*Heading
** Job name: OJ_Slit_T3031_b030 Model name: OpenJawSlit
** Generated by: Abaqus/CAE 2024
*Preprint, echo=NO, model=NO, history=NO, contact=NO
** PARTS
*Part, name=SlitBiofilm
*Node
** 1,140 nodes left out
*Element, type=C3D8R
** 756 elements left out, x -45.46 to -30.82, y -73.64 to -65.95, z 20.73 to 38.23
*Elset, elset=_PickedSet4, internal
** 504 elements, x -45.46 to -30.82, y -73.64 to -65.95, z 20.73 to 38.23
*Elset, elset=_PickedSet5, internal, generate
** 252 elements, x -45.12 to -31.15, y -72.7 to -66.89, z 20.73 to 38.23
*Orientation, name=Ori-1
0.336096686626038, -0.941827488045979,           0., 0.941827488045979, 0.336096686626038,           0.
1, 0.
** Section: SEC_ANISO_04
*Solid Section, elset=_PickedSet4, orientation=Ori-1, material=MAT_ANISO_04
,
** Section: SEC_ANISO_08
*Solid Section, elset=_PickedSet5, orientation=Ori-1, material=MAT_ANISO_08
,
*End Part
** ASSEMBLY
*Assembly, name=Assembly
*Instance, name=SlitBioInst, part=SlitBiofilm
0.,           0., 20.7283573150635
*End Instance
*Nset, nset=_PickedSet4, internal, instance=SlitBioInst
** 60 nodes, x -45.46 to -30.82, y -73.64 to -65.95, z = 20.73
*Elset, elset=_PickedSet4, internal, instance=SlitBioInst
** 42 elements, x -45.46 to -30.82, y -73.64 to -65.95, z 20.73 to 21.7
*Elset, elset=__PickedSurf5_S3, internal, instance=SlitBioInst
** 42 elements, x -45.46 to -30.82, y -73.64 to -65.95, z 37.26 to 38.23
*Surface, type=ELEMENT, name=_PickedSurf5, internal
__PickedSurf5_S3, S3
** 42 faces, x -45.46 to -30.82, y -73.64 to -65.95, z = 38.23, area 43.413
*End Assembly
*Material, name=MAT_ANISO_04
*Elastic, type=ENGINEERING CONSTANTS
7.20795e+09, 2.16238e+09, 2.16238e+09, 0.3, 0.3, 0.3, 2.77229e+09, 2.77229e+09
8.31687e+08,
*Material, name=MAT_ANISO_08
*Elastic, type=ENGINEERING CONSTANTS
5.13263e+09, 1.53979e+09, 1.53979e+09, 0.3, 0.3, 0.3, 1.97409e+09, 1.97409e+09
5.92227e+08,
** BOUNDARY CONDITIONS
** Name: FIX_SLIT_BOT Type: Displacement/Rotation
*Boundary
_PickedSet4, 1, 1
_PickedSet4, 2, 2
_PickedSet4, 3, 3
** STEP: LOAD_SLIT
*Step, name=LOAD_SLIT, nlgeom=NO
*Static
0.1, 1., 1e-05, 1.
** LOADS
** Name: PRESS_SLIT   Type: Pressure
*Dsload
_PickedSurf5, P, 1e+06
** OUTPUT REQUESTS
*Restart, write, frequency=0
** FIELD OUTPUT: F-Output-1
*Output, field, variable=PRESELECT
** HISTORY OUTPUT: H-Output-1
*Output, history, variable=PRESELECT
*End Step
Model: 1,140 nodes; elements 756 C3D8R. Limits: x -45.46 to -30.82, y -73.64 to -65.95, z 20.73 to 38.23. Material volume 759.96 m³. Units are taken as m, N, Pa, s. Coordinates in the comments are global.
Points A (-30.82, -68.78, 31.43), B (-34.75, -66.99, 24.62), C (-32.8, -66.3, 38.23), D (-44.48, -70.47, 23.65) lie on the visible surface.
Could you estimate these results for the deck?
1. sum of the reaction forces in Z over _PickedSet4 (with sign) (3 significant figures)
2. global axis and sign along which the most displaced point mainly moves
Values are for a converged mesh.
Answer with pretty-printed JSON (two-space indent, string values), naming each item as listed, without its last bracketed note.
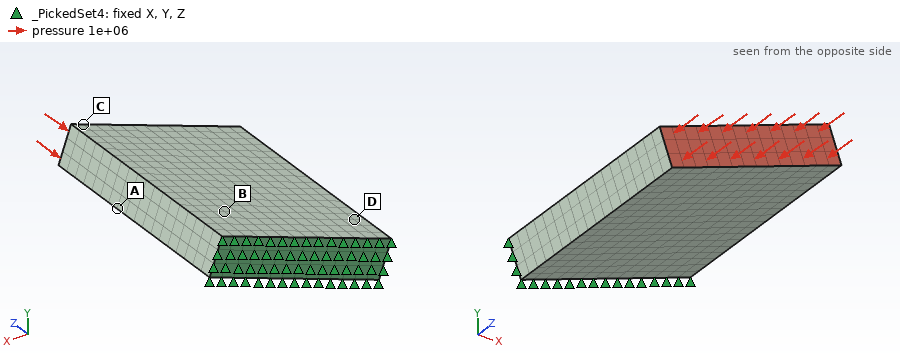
{
  "sum of the reaction forces in Z over _PickedSet4 (with sign)": "4.34e+07 N",
  "global axis and sign along which the most displaced point mainly moves": "-Z"
}
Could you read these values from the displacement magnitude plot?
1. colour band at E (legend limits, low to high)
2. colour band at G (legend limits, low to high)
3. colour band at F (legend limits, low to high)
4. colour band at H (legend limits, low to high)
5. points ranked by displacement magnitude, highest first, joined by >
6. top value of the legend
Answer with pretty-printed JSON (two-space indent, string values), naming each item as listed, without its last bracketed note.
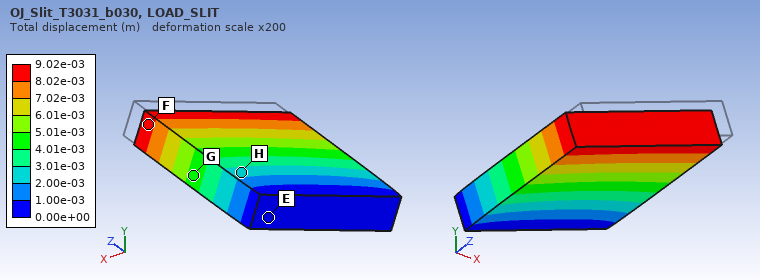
{
  "colour band at E": "0.00e+00 to 1.00e-03 m",
  "colour band at G": "4.01e-03 to 5.01e-03 m",
  "colour band at F": "8.02e-03 to 9.02e-03 m",
  "colour band at H": "2.00e-03 to 3.01e-03 m",
  "points ranked by displacement magnitude, highest first, joined by >": "F > G > H > E",
  "top value of the legend": "9.02e-03 m"
}
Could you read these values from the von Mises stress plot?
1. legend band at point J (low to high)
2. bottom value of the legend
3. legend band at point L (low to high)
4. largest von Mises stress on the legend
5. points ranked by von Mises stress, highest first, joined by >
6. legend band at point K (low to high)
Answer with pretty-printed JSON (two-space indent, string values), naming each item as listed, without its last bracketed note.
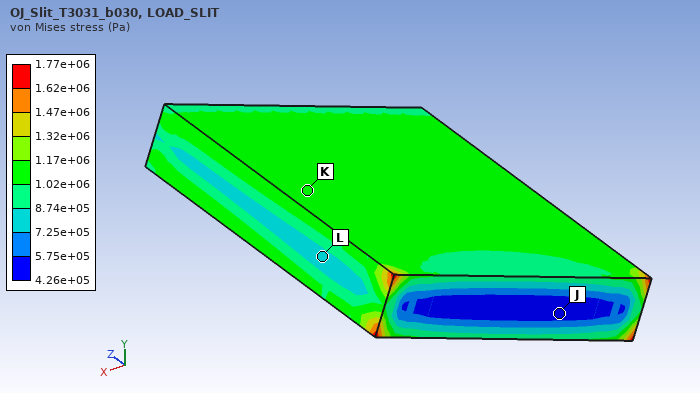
{
  "legend band at point J": "4.26e+05 to 5.75e+05 Pa",
  "bottom value of the legend": "4.26e+05 Pa",
  "legend band at point L": "7.25e+05 to 8.74e+05 Pa",
  "largest von Mises stress on the legend": "1.77e+06 Pa",
  "points ranked by von Mises stress, highest first, joined by >": "K > L > J",
  "legend band at point K": "1.02e+06 to 1.17e+06 Pa"
}
